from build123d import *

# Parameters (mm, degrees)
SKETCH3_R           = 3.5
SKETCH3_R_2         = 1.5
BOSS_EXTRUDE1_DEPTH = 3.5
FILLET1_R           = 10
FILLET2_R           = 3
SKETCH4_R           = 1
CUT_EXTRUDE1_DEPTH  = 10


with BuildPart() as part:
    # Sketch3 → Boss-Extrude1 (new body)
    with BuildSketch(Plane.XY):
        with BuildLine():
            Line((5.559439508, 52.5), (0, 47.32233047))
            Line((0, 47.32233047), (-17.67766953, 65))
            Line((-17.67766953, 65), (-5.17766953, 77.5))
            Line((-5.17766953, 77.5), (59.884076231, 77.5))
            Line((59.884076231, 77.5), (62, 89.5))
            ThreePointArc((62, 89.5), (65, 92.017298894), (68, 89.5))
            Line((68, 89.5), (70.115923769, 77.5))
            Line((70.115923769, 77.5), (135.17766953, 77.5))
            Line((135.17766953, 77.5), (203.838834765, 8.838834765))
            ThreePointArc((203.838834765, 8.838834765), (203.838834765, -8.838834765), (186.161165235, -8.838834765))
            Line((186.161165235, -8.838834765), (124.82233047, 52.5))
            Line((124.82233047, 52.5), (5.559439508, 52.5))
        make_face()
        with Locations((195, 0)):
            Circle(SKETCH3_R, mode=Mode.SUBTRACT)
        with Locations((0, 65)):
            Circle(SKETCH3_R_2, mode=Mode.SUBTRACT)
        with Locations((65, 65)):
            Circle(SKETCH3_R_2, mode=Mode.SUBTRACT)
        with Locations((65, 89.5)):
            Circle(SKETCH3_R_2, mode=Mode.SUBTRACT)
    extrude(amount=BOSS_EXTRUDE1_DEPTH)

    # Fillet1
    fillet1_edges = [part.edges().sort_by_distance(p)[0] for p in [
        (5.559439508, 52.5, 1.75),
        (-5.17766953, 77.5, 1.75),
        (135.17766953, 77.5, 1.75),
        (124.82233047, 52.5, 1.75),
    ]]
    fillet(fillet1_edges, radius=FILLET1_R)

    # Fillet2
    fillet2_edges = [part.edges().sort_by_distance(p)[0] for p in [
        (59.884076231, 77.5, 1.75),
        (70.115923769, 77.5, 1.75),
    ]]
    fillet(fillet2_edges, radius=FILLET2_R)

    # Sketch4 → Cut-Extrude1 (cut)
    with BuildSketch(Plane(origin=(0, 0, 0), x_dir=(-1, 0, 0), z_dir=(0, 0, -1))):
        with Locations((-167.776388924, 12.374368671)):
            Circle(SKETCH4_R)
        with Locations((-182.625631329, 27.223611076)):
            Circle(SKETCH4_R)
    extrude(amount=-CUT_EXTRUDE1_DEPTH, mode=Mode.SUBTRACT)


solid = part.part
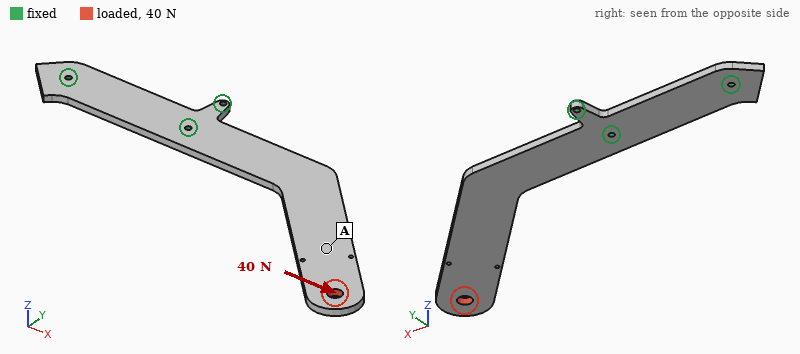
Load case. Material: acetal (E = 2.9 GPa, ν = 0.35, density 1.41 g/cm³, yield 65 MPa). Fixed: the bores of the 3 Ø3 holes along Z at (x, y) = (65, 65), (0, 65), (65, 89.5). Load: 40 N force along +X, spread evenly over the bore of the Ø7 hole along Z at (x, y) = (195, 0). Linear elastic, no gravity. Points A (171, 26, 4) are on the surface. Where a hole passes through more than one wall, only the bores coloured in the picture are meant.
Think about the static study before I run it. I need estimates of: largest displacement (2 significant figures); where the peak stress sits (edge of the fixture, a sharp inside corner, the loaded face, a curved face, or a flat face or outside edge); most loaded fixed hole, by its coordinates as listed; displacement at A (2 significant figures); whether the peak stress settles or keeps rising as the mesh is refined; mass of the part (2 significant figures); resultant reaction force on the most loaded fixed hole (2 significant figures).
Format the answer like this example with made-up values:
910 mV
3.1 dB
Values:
2.7 mm
edge of the fixture
(65, 65)
1.5 mm
keeps rising
30 g
72 N
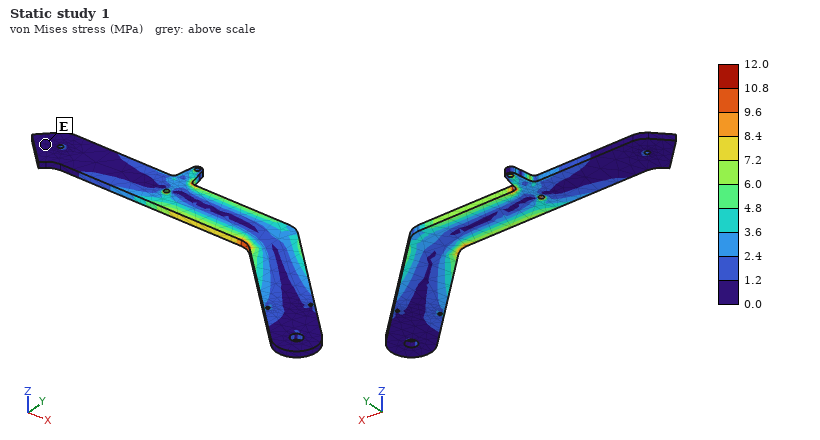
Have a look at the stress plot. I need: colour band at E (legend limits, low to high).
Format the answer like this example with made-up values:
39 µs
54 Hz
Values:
0.0 to 1.2 MPa
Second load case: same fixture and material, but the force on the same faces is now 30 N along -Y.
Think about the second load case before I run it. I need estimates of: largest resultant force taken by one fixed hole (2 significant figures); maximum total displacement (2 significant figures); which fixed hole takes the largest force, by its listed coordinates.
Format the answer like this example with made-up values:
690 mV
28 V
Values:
83 N
2.9 mm
(65, 89.5)
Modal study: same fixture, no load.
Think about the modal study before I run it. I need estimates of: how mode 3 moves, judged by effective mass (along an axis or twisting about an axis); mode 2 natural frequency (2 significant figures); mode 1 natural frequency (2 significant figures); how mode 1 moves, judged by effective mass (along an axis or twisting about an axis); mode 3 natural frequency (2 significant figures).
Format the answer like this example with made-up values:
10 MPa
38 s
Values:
along Y
160 Hz
33 Hz
along Z
200 Hz
